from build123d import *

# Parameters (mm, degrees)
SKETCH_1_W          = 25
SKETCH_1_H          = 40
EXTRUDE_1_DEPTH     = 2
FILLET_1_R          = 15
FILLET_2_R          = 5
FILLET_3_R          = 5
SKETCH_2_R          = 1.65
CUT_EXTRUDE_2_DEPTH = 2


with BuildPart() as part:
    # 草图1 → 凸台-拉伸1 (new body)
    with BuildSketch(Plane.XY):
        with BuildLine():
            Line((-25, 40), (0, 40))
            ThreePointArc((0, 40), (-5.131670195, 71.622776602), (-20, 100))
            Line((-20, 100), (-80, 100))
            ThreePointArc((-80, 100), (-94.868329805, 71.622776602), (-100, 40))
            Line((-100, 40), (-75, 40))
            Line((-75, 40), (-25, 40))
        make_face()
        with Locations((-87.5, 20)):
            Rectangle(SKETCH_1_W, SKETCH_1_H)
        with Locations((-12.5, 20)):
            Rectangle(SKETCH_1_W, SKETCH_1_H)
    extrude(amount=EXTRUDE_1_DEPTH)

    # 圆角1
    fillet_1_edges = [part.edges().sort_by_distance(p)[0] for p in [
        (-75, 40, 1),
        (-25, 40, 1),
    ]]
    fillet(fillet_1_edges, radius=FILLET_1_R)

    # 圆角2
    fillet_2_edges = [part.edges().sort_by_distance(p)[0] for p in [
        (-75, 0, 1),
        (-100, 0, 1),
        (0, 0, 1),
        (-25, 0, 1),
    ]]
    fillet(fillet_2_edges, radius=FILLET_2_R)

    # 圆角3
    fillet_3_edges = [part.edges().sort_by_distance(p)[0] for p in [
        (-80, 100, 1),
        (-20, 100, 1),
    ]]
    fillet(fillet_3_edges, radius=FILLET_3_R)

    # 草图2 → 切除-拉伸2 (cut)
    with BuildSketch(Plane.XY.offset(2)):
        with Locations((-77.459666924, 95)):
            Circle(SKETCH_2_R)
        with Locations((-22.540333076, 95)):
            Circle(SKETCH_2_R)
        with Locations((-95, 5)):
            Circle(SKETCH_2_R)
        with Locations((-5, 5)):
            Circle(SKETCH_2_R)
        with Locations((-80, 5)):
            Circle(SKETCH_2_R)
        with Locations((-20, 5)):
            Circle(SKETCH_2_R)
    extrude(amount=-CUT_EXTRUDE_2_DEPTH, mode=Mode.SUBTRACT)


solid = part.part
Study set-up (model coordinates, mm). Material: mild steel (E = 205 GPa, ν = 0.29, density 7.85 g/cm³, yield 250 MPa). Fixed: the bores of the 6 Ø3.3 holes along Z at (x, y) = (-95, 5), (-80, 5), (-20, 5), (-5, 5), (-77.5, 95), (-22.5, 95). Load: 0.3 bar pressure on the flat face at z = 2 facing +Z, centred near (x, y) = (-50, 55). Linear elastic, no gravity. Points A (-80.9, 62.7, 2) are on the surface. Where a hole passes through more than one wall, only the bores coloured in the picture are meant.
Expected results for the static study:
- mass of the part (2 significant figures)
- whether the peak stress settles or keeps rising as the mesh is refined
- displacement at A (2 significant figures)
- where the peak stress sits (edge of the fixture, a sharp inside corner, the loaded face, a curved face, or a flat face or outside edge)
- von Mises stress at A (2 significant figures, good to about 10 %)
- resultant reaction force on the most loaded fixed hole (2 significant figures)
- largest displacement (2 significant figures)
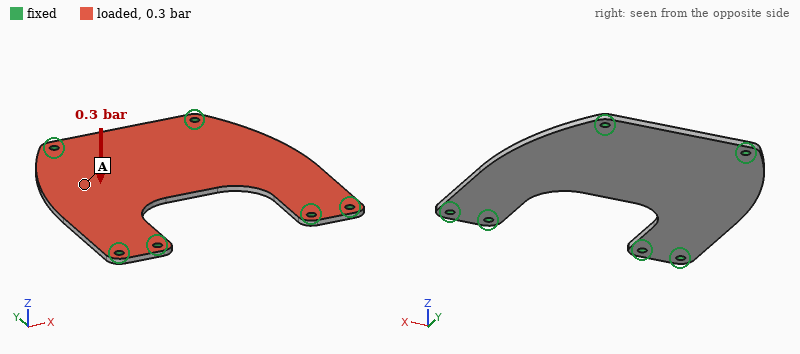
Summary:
110 g
keeps rising
45 µm
edge of the fixture
15 MPa
60 N
66 µm
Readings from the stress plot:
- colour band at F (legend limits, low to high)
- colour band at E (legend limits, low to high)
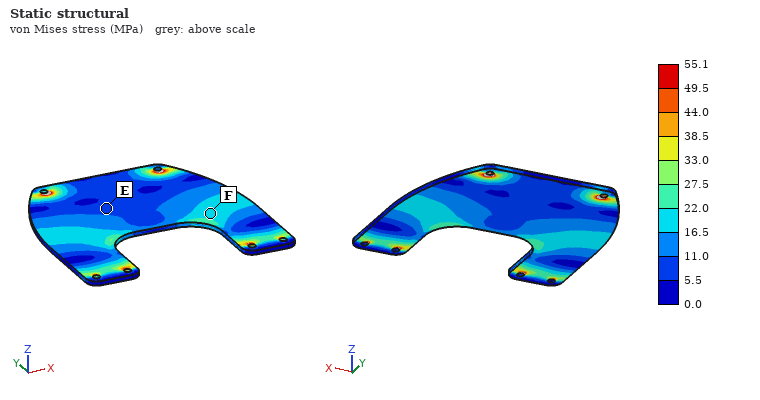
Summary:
16.5 to 22.0 MPa
5.5 to 11.0 MPa
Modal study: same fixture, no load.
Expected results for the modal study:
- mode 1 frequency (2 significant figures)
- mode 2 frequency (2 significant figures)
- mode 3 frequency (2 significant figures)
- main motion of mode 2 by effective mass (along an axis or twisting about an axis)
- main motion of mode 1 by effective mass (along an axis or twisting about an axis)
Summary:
1000 Hz
1300 Hz
1900 Hz
twisting about Y
along Z
